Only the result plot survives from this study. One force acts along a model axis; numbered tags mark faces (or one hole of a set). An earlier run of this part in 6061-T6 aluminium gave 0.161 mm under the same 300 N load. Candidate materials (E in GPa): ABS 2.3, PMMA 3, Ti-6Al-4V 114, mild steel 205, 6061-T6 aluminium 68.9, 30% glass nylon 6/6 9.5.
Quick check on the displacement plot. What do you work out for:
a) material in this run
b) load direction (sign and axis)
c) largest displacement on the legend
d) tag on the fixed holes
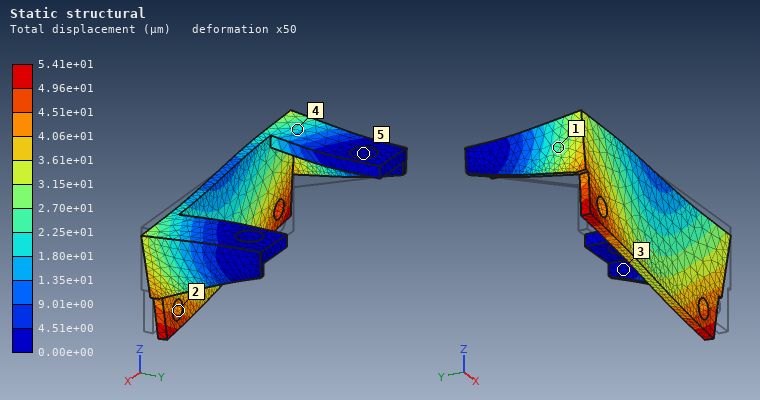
mild steel
-X
5.41e+01 µm
5
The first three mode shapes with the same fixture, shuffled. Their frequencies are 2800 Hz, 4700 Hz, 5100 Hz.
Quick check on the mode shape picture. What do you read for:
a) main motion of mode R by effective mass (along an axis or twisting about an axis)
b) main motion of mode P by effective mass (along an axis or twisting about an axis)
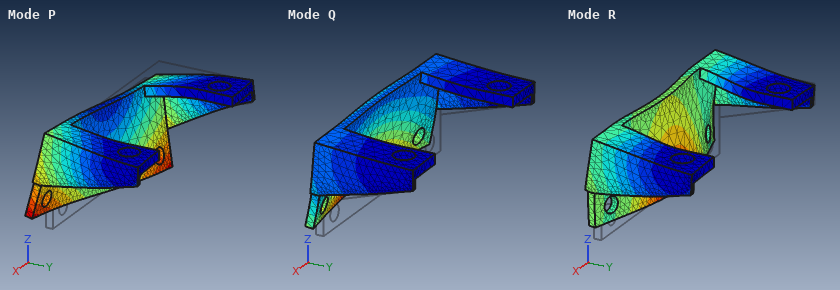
along Z
along X
